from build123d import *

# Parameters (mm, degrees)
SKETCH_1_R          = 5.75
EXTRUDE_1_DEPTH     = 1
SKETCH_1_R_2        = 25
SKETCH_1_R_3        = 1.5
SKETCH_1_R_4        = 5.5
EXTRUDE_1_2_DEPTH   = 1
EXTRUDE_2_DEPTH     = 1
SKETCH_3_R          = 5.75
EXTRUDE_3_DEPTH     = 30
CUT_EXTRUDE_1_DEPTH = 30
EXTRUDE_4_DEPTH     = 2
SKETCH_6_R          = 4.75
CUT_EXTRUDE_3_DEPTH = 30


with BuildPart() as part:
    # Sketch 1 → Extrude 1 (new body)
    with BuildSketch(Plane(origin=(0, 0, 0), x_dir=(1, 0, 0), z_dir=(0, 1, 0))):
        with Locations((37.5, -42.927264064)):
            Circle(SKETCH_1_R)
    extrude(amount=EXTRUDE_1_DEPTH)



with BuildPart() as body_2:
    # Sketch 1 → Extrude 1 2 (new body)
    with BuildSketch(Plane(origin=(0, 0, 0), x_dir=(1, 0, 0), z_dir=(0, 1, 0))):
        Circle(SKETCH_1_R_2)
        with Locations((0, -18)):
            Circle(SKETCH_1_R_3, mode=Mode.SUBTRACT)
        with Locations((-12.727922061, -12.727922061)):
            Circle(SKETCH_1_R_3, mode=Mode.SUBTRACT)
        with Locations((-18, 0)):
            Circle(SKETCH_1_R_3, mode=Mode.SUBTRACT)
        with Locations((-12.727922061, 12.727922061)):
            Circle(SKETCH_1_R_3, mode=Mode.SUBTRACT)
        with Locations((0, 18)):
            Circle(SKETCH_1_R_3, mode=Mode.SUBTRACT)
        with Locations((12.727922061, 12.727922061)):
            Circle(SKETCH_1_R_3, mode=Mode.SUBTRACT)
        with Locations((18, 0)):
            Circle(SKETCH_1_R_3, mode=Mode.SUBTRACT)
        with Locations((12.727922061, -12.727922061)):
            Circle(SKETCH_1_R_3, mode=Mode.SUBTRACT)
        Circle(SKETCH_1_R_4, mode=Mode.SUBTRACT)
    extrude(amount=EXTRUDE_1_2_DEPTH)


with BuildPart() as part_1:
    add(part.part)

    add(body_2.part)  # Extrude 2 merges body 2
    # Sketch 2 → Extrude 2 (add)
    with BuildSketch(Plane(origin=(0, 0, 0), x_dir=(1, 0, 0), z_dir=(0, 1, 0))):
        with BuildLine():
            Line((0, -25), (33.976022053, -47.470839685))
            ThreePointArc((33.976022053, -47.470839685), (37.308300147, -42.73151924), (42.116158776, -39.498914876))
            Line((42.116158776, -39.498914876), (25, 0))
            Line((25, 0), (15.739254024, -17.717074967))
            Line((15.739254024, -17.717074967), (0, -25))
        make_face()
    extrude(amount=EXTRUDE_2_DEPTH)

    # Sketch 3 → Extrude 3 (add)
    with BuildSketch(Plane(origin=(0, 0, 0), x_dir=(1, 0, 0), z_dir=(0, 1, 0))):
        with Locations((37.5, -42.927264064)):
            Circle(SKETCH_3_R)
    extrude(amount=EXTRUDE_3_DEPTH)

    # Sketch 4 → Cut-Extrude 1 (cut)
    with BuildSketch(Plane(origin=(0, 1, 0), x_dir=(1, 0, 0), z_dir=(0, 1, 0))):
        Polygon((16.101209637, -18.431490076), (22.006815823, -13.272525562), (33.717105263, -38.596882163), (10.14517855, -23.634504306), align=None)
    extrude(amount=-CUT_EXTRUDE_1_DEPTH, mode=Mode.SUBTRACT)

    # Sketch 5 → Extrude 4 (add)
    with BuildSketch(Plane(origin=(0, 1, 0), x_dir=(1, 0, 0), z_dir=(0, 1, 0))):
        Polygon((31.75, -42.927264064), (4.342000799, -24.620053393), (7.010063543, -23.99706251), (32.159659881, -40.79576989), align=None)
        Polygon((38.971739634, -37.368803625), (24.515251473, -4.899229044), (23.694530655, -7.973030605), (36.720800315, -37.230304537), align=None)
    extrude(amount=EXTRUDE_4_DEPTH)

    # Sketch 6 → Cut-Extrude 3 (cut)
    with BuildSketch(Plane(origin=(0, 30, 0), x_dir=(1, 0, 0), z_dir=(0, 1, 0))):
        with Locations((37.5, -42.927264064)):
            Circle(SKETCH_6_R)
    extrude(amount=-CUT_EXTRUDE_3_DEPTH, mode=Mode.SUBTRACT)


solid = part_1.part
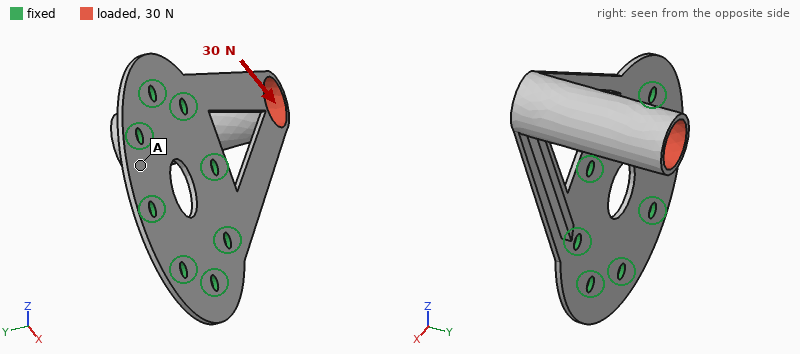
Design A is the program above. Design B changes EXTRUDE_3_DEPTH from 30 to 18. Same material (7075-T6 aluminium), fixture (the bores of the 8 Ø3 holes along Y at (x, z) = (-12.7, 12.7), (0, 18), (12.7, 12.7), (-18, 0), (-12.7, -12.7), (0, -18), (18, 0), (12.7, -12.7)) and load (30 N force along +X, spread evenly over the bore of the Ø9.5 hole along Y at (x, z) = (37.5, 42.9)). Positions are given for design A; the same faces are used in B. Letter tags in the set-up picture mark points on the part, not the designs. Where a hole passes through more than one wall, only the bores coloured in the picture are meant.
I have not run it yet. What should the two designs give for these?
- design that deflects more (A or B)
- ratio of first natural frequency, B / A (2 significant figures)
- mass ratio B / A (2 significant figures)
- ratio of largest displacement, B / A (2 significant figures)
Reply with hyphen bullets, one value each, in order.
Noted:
- A
- 1.3
- 0.89
- 0.46
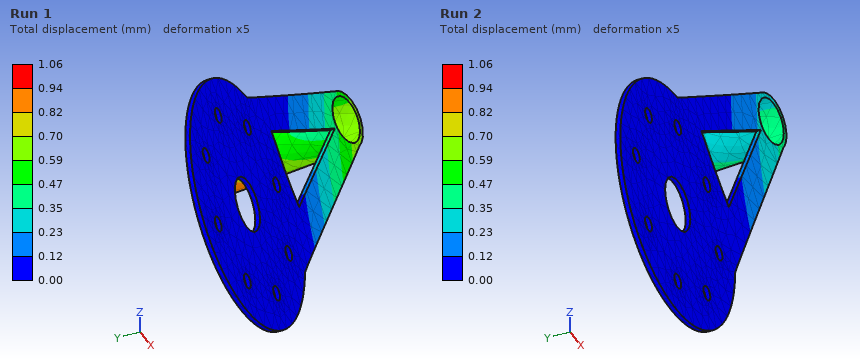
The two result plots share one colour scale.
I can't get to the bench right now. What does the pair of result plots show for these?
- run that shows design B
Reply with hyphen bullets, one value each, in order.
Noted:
- Run 2
